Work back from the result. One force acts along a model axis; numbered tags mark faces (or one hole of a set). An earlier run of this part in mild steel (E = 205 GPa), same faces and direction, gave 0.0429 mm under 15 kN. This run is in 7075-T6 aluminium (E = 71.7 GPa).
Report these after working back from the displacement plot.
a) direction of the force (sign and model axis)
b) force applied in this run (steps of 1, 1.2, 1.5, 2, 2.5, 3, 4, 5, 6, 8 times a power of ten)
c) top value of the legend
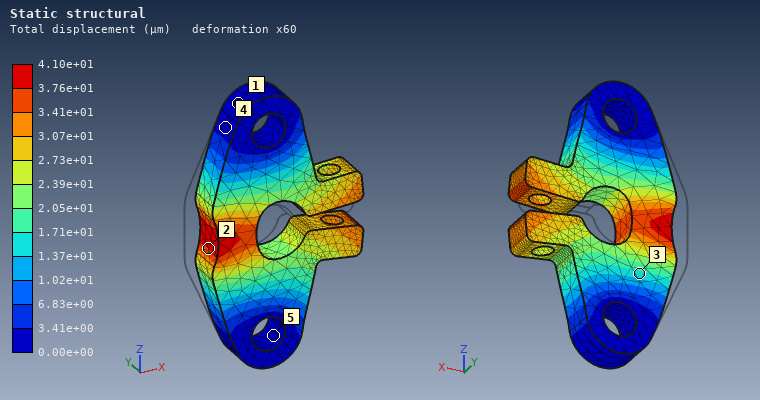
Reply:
+X
5 kN
4.10e+01 µm
